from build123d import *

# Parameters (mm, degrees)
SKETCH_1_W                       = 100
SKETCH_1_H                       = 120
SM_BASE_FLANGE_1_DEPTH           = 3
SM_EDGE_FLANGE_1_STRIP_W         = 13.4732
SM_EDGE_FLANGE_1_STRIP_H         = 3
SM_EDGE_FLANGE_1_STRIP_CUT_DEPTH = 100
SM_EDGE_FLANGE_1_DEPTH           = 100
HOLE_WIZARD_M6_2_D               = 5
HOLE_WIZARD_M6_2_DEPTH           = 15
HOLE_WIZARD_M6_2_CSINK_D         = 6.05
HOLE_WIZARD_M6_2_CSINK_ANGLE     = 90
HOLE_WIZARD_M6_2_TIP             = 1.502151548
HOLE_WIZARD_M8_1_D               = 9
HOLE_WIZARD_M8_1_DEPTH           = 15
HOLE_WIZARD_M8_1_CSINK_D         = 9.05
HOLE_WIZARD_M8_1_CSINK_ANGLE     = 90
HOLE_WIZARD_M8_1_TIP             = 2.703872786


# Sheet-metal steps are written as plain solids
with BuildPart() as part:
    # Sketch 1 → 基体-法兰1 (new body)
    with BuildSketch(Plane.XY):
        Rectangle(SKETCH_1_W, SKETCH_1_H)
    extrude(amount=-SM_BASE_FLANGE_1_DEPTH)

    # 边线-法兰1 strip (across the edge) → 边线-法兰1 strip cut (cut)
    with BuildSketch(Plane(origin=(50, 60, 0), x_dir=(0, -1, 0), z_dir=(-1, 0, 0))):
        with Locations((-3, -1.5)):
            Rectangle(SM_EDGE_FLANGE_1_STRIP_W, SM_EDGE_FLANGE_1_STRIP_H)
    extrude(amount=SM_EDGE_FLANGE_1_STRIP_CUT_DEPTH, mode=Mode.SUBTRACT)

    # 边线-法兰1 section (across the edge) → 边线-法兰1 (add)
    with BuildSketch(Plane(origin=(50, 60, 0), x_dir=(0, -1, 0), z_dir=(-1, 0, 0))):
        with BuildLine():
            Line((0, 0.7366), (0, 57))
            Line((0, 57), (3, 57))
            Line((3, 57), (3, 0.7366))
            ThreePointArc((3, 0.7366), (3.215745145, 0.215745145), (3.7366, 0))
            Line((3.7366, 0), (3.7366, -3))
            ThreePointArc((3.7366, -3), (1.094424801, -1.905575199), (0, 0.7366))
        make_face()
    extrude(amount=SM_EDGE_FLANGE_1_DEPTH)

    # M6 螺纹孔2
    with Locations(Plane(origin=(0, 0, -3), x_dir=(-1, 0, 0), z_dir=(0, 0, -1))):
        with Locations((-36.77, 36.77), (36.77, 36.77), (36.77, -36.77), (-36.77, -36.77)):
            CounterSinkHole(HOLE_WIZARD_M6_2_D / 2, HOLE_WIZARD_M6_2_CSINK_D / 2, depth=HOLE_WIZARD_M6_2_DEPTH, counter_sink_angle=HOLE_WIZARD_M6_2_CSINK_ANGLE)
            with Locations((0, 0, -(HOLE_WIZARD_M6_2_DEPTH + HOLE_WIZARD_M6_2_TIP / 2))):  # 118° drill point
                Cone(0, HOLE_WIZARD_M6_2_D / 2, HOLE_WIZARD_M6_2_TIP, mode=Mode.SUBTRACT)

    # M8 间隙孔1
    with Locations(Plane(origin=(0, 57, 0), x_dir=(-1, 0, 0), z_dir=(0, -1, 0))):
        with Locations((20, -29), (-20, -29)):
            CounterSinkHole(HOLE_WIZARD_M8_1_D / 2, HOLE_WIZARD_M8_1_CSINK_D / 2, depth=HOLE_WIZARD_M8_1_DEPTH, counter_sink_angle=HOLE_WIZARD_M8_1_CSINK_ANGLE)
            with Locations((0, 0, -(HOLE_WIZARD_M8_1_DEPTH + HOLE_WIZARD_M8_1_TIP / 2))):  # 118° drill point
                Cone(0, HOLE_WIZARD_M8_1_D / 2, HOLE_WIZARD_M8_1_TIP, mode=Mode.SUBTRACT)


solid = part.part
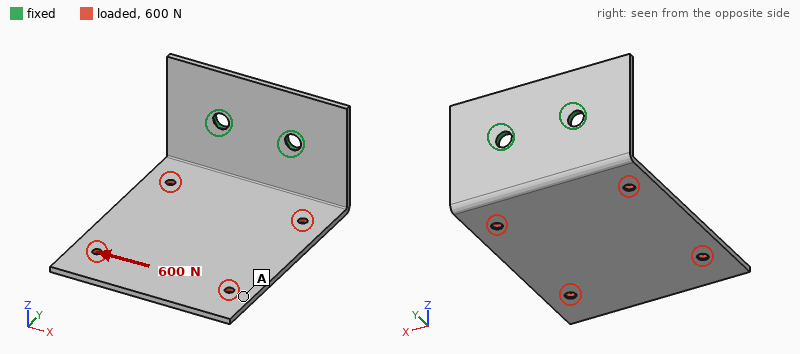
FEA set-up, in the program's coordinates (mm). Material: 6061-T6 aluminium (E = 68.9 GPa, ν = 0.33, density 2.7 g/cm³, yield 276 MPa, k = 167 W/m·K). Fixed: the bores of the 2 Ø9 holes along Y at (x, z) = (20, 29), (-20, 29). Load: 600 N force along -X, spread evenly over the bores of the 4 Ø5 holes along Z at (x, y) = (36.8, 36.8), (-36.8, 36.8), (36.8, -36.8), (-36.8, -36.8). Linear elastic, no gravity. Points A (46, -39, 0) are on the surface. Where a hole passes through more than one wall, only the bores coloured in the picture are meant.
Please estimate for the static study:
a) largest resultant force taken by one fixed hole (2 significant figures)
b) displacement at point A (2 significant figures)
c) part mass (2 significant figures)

810 N
1.7 mm
140 g
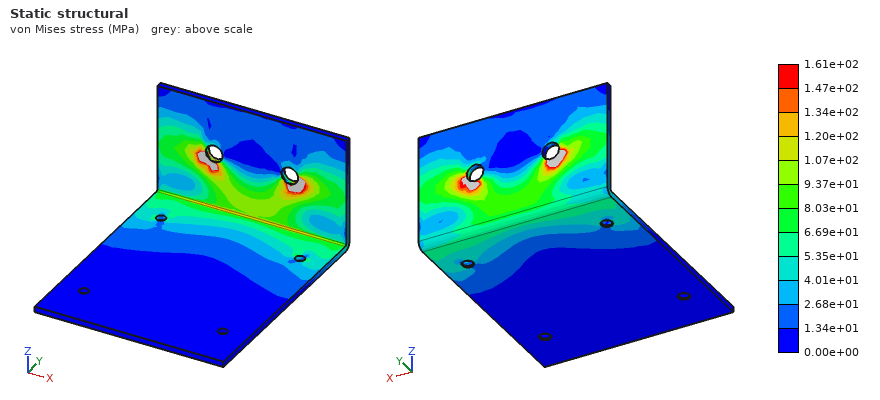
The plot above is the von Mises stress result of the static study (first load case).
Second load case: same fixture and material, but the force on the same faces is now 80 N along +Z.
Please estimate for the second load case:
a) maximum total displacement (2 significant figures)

2.0 mm
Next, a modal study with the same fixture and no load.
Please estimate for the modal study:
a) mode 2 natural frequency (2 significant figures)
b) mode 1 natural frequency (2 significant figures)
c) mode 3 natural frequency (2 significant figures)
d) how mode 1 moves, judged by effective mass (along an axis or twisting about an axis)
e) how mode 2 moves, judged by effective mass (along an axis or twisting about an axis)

320 Hz
130 Hz
490 Hz
along Z
along X
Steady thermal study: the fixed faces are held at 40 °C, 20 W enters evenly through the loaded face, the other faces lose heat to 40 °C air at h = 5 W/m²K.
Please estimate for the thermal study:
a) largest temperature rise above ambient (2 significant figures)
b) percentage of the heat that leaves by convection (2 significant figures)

34 K
16 %
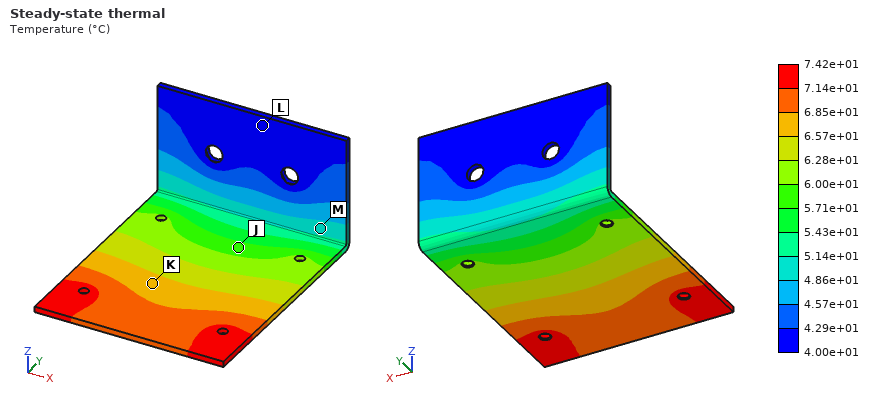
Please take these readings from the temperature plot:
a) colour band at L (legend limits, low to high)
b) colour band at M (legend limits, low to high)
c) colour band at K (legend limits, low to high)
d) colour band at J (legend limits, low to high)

4.00e+01 to 4.29e+01 °C
4.86e+01 to 5.14e+01 °C
6.57e+01 to 6.85e+01 °C
5.71e+01 to 6.00e+01 °C
